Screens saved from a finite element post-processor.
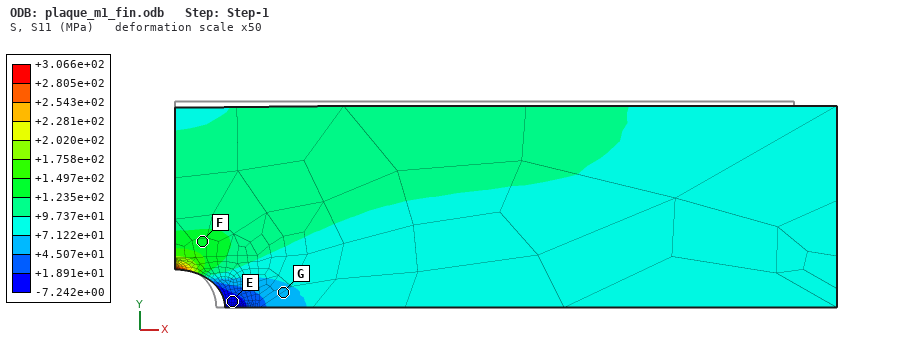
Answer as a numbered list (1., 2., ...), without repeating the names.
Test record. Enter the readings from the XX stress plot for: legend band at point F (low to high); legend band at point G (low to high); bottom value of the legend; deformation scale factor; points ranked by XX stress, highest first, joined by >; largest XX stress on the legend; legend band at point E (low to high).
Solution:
1. +1.235e+02 to +1.497e+02 MPa
2. +4.507e+01 to +7.122e+01 MPa
3. -7.242e+00 MPa
4. 50
5. F > G > E
6. +3.066e+02 MPa
7. -7.242e+00 to +1.891e+01 MPa
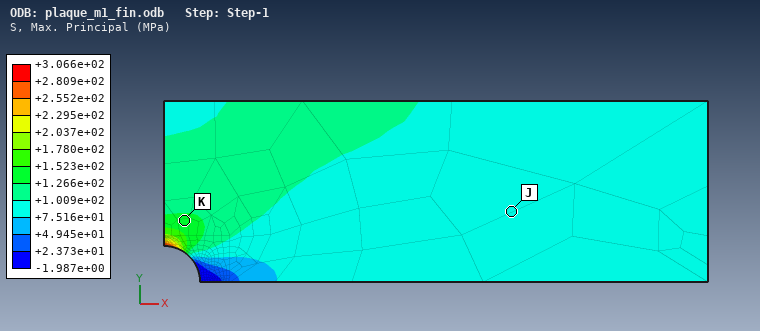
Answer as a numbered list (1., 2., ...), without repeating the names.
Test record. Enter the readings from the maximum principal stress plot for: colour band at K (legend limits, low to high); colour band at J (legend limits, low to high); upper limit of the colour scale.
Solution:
1. +1.266e+02 to +1.523e+02 MPa
2. +7.516e+01 to +1.009e+02 MPa
3. +3.066e+02 MPa
